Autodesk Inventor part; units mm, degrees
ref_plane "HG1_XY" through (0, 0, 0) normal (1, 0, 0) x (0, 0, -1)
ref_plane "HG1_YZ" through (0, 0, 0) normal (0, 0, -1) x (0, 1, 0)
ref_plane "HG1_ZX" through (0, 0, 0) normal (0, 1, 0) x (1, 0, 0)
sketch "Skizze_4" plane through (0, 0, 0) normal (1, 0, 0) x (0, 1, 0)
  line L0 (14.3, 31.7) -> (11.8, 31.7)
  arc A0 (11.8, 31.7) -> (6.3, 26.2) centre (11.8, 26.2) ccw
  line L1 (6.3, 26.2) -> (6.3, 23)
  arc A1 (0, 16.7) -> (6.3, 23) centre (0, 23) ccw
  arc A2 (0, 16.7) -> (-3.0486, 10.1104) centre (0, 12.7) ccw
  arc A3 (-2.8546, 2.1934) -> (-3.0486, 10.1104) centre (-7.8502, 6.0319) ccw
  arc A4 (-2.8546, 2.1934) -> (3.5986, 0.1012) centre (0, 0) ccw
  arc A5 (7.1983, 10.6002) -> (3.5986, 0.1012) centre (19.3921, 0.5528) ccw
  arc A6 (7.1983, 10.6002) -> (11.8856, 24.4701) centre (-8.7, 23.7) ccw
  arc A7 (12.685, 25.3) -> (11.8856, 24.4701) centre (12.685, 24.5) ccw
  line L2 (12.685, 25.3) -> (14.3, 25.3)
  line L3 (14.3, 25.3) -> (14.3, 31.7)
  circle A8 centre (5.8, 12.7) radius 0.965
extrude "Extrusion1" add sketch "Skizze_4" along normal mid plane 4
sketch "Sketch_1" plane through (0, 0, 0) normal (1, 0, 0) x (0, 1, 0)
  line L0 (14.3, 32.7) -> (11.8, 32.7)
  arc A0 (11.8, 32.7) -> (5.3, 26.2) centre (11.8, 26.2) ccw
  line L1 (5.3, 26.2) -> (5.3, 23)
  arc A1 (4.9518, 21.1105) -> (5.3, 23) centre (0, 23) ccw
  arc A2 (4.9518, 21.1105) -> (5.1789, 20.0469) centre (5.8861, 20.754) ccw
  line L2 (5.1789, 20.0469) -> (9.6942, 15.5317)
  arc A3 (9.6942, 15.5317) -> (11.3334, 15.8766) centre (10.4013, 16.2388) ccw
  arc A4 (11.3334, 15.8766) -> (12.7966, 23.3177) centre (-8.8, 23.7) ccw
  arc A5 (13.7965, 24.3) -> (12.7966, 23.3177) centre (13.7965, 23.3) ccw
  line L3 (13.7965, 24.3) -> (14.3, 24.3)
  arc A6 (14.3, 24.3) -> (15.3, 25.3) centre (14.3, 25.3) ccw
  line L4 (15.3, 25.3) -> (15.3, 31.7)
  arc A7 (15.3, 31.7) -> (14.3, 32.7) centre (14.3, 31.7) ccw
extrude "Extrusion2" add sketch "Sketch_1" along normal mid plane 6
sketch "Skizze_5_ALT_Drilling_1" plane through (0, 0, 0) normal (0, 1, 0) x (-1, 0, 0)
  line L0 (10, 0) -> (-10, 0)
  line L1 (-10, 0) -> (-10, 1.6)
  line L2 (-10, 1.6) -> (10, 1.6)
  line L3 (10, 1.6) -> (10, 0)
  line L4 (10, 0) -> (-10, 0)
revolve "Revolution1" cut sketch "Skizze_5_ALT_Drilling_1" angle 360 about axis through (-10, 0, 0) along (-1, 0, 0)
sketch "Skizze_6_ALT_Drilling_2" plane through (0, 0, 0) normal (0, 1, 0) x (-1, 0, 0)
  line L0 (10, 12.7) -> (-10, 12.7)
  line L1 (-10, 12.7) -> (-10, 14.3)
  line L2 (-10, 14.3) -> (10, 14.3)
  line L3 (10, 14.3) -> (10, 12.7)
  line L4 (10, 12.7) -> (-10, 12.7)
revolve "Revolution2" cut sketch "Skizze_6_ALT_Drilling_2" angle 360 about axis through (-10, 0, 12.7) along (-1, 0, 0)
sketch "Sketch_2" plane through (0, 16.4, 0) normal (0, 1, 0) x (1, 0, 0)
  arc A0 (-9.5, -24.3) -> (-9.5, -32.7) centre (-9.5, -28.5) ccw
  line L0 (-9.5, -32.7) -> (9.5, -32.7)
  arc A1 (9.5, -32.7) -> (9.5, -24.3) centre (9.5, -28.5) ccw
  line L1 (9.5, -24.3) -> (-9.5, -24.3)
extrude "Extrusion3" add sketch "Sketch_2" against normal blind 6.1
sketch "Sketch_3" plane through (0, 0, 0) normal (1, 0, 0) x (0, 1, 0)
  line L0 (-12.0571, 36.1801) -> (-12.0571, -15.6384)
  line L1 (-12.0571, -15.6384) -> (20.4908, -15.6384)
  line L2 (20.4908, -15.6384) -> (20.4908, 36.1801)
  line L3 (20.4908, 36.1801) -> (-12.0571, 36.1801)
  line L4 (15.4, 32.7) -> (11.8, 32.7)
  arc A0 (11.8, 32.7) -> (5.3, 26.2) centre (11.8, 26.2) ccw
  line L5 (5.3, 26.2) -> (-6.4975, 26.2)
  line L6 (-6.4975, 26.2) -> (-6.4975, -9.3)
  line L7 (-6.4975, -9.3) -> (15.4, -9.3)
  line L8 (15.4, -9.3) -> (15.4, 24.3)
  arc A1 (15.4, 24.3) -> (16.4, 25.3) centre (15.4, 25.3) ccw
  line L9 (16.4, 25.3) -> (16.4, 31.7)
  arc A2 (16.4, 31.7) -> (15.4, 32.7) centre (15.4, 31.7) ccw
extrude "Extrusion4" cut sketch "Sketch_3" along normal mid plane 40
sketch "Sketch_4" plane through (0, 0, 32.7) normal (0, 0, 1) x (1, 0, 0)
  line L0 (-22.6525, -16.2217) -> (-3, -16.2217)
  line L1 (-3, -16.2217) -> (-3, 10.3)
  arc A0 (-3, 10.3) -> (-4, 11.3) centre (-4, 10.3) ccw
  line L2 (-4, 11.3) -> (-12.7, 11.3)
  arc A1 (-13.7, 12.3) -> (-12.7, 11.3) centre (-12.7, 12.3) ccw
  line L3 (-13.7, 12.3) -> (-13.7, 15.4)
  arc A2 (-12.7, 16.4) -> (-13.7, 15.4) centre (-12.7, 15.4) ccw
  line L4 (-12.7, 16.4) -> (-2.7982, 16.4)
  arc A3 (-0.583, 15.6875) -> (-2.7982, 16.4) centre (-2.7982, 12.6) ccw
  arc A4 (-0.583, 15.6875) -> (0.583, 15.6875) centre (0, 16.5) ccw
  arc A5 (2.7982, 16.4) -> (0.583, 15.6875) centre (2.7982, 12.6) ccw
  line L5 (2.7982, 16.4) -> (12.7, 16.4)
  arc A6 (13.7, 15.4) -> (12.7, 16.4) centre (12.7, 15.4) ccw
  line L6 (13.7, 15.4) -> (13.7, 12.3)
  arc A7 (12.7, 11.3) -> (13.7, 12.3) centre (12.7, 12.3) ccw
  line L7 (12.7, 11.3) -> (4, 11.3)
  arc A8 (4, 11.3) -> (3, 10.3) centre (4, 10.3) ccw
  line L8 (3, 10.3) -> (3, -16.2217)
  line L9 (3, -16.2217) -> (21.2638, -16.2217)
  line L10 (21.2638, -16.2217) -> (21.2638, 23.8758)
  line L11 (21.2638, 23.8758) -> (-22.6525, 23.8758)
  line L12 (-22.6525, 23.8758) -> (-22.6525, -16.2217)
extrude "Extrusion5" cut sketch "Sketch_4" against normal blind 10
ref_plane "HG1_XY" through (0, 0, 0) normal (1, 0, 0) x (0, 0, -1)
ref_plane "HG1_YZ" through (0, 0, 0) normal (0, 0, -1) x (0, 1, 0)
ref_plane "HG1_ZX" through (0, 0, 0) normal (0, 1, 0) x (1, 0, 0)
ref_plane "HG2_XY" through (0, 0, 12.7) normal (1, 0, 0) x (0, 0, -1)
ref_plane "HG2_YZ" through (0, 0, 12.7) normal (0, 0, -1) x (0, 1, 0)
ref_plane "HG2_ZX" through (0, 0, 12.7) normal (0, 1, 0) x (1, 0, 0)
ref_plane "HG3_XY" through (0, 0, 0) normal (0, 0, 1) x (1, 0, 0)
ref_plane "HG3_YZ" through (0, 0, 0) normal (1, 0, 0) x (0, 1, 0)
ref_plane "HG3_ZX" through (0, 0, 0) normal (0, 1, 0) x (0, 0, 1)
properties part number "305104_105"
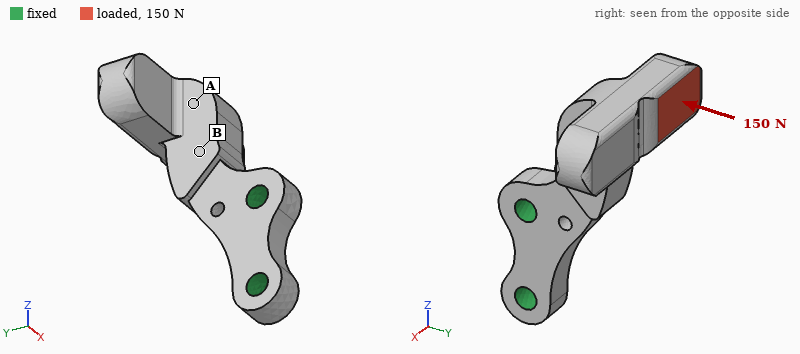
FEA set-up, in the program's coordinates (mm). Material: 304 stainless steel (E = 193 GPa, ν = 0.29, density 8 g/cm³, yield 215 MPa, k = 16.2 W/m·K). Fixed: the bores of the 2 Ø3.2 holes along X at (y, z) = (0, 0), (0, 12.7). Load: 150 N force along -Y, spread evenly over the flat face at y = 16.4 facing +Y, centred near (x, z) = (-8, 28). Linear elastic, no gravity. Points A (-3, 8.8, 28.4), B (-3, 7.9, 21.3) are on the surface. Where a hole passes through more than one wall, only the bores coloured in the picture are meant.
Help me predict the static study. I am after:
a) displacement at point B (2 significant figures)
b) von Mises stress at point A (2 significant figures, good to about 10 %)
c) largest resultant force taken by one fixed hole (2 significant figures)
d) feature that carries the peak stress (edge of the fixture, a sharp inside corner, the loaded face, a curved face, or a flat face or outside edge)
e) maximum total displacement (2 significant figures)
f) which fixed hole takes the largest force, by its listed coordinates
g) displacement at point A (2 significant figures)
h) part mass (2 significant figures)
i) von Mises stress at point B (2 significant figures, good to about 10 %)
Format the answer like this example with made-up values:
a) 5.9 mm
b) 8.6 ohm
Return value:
a) 11 µm
b) 18 MPa
c) 310 N
d) a curved face
e) 49 µm
f) (0, 12.7)
g) 19 µm
h) 18 g
i) 44 MPa
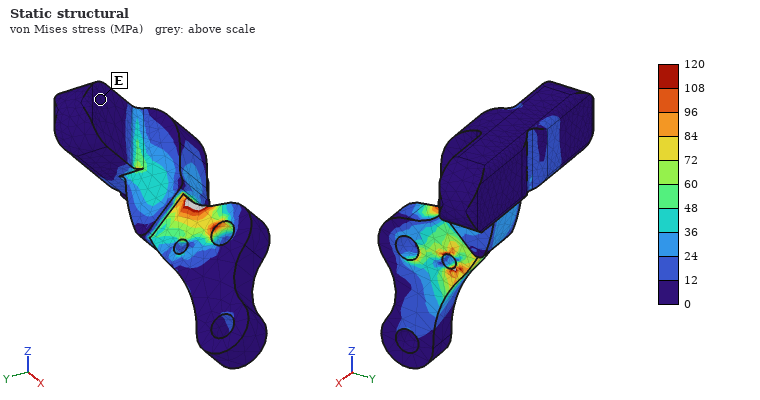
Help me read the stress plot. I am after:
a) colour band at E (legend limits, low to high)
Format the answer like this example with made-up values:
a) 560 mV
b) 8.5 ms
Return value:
a) 0 to 12 MPa
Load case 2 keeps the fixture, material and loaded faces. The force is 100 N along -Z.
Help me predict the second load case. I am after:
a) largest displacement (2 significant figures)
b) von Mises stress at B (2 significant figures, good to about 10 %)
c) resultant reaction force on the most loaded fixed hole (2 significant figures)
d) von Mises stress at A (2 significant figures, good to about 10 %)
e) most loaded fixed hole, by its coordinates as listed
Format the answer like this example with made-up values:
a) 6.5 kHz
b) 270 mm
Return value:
a) 30 µm
b) 17 MPa
c) 140 N
d) 6.8 MPa
e) (0, 0)
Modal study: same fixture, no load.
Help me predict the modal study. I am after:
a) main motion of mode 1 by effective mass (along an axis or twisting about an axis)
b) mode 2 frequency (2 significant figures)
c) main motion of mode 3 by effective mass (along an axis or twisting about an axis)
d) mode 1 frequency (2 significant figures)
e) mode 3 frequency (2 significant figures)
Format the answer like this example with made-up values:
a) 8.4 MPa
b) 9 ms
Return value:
a) along X
b) 4400 Hz
c) twisting about Z
d) 2400 Hz
e) 5300 Hz
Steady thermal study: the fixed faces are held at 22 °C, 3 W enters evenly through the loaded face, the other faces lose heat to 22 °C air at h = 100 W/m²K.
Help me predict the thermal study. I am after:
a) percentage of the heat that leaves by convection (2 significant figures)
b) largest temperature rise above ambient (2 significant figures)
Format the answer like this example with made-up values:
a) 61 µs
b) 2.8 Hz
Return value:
a) 81 %
b) 49 K
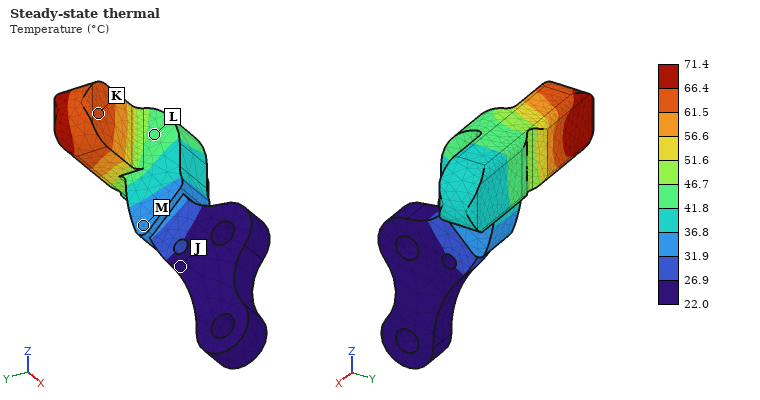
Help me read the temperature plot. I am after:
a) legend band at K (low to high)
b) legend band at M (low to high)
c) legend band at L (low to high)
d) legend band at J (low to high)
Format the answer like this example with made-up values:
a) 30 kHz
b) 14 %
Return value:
a) 61.5 to 66.4 °C
b) 31.9 to 36.8 °C
c) 41.8 to 46.7 °C
d) 22.0 to 26.9 °C
